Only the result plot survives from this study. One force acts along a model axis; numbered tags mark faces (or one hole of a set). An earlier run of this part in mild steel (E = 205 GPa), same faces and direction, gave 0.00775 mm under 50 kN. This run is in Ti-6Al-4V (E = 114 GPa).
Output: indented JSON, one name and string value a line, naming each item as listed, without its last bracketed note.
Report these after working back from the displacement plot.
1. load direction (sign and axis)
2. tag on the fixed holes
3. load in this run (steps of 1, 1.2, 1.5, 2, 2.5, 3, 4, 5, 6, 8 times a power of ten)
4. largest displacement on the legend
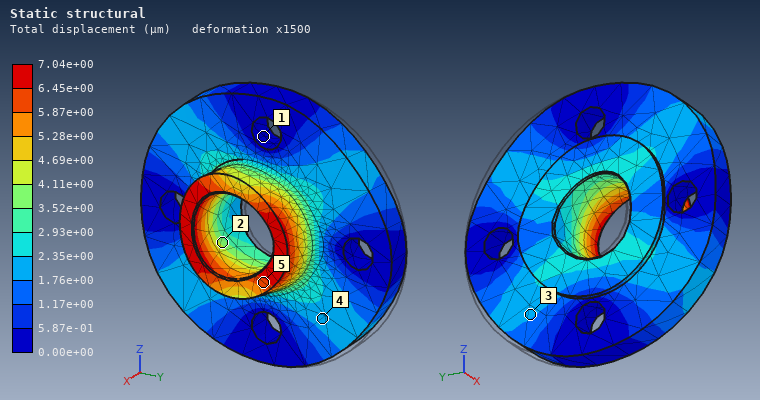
{
  "load direction": "-Y",
  "tag on the fixed holes": "1",
  "load in this run": "25 kN",
  "largest displacement on the legend": "7.04e+00 µm"
}
